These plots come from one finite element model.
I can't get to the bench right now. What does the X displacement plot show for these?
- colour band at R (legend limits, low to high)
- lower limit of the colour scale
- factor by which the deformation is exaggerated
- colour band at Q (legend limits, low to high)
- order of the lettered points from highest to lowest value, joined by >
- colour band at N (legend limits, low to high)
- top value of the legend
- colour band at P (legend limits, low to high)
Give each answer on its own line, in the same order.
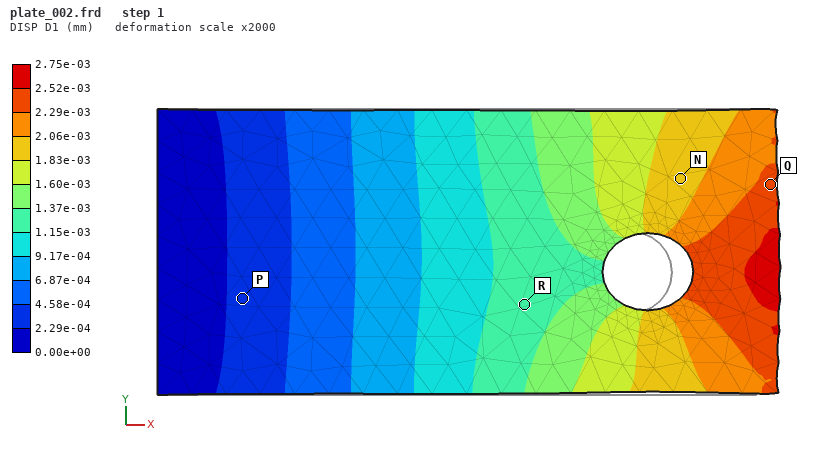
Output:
1.15e-03 to 1.37e-03 mm
0.00e+00 mm
2000
2.29e-03 to 2.52e-03 mm
Q > N > R > P
1.83e-03 to 2.06e-03 mm
2.75e-03 mm
2.29e-04 to 4.58e-04 mm
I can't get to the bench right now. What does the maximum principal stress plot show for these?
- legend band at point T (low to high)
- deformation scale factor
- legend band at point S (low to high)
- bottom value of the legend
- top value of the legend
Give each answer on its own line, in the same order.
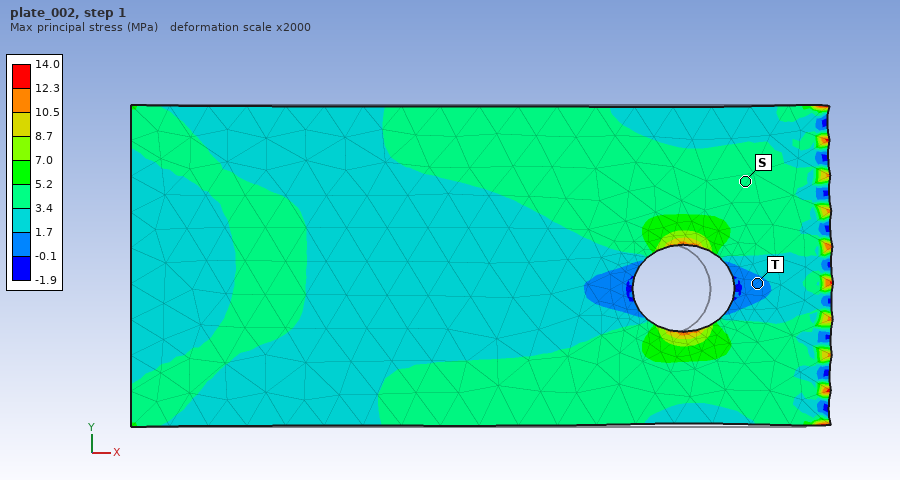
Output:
-0.1 to 1.7 MPa
2000
3.4 to 5.2 MPa
-1.9 MPa
14.0 MPa
